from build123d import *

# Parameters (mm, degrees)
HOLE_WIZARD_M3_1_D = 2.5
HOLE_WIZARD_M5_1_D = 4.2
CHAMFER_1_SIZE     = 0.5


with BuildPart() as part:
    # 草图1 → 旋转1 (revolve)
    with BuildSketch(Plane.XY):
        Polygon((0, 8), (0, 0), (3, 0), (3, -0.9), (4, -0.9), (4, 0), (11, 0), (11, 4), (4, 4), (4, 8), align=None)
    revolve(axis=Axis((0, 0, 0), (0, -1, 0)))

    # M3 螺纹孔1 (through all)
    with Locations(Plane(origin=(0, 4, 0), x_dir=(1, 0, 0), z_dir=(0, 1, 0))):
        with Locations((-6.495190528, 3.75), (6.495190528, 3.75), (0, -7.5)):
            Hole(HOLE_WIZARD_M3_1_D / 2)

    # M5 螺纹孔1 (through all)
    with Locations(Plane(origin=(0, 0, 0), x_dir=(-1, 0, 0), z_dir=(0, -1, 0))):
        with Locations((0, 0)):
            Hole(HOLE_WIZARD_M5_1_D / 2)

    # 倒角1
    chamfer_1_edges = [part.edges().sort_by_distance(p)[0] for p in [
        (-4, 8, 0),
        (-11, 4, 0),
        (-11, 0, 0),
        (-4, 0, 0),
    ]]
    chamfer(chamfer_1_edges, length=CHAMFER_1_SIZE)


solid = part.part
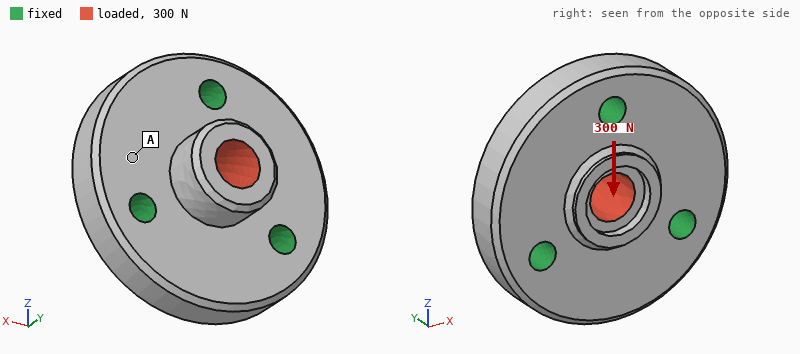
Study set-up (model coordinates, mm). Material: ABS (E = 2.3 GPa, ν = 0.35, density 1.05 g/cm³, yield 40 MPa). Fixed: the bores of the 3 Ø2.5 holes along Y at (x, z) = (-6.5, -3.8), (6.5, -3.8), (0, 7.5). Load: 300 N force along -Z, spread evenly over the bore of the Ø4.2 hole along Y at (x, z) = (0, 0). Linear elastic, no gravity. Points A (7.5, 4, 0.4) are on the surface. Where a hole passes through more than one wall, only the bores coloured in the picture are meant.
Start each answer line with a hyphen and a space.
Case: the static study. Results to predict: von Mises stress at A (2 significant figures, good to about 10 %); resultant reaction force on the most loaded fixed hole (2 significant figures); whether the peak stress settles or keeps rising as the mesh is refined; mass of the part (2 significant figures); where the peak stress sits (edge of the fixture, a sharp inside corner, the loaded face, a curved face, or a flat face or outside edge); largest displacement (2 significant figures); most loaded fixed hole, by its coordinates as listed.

- 1.7 MPa
- 120 N
- keeps rising
- 1.6 g
- edge of the fixture
- 51 µm
- (0, 7.5)
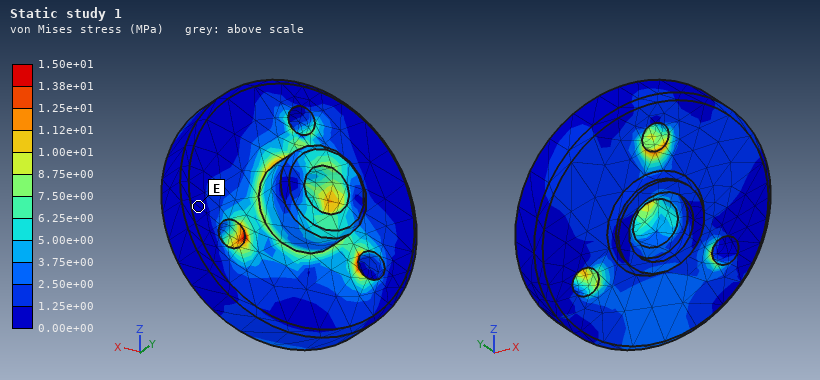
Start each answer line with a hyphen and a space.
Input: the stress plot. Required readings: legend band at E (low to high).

- 0.00e+00 to 1.25e+00 MPa
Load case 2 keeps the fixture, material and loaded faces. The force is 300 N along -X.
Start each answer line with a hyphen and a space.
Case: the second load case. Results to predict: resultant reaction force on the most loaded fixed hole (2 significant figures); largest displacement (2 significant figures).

- 110 N
- 49 µm
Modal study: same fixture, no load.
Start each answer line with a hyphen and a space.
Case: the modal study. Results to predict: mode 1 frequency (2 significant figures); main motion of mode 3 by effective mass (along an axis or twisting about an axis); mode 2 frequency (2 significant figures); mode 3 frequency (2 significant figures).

- 16 kHz
- along Y
- 16 kHz
- 18 kHz
